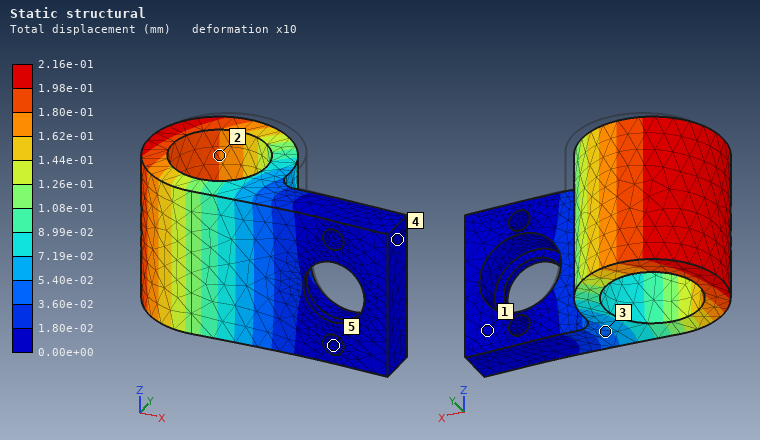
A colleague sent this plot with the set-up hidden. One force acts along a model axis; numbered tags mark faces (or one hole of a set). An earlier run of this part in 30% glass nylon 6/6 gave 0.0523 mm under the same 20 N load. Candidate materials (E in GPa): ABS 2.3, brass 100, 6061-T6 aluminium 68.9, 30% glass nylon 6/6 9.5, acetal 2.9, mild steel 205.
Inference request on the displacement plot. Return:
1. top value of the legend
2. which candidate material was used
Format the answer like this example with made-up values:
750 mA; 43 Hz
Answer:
2.16e-01 mm; ABS
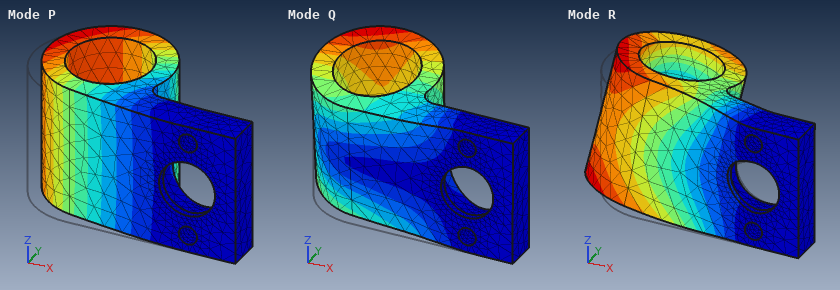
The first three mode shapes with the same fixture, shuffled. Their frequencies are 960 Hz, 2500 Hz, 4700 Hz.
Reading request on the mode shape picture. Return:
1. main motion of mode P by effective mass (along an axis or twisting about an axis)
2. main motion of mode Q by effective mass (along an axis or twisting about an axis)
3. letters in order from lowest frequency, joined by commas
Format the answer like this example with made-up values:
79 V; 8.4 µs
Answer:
along Y; along Z; P, Q, R
